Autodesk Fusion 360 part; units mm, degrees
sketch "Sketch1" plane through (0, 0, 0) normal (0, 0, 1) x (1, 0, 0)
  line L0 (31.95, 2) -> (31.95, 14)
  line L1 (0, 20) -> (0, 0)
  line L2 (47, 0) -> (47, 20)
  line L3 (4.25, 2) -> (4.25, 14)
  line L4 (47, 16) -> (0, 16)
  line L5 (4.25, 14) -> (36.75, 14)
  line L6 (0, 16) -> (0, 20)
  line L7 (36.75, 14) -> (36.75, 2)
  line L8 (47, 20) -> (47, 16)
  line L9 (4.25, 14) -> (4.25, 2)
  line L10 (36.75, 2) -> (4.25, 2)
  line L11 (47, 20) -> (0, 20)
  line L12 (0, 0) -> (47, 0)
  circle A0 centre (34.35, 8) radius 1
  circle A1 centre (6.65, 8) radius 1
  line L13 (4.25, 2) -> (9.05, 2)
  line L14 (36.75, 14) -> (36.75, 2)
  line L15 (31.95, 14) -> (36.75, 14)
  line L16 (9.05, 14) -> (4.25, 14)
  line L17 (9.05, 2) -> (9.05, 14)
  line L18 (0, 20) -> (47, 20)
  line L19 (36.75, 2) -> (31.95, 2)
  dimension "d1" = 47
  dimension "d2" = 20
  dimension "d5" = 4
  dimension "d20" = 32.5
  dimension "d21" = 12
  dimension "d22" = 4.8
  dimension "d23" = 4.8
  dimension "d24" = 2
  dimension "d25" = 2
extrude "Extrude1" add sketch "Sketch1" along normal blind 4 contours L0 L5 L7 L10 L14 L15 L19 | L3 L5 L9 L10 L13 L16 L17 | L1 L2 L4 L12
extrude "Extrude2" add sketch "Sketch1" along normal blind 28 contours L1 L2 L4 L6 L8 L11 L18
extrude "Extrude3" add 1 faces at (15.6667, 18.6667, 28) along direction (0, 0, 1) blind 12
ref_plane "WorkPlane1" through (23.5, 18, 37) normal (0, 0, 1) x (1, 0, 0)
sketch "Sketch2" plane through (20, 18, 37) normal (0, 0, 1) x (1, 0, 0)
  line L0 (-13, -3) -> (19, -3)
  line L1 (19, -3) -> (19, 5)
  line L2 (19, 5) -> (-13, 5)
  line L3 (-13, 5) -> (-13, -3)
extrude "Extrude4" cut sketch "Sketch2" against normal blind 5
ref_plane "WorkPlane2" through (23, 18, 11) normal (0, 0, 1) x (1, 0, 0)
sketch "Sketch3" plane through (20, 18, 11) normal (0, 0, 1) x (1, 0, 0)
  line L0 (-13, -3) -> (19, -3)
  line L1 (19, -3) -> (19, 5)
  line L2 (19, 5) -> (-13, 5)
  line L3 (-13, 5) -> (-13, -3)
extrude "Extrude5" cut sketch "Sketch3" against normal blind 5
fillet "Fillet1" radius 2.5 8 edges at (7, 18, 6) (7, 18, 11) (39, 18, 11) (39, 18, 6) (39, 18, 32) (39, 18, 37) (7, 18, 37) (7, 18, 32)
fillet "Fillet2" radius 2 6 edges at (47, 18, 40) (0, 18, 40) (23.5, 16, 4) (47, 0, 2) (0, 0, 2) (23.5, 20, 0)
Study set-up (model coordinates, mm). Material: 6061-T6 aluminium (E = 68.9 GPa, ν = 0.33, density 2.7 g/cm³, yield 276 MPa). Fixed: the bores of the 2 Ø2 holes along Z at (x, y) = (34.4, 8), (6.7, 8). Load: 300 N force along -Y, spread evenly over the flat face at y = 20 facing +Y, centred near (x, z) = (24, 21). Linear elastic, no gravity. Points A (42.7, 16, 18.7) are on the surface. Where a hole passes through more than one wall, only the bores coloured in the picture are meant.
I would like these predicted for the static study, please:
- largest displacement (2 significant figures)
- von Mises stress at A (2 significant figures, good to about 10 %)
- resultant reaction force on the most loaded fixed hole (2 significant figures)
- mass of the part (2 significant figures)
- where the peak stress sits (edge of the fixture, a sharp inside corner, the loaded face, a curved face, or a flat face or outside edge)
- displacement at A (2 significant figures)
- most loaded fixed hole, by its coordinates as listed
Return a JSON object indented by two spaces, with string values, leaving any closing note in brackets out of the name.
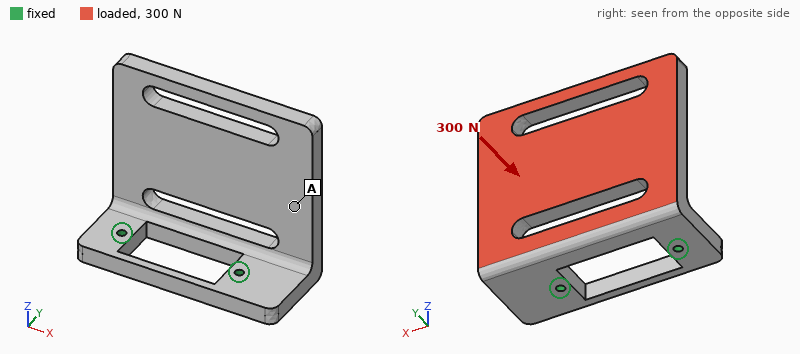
{
  "largest displacement": "0.52 mm",
  "von Mises stress at A": "25 MPa",
  "resultant reaction force on the most loaded fixed hole": "170 N",
  "mass of the part": "22 g",
  "where the peak stress sits": "a flat face or outside edge",
  "displacement at A": "0.18 mm",
  "most loaded fixed hole, by its coordinates as listed": "(34.4, 8)"
}
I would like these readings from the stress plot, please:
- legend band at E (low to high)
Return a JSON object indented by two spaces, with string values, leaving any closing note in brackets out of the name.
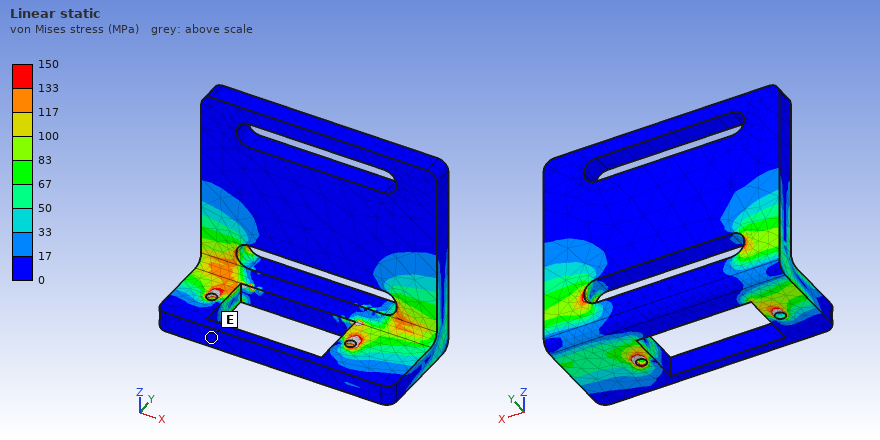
{
  "legend band at E": "0 to 17 MPa"
}
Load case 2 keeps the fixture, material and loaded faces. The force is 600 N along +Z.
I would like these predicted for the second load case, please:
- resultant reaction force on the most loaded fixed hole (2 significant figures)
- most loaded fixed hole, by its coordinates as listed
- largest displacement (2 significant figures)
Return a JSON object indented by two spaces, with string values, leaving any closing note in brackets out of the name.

{
  "resultant reaction force on the most loaded fixed hole": "350 N",
  "most loaded fixed hole, by its coordinates as listed": "(34.4, 8)",
  "largest displacement": "0.31 mm"
}
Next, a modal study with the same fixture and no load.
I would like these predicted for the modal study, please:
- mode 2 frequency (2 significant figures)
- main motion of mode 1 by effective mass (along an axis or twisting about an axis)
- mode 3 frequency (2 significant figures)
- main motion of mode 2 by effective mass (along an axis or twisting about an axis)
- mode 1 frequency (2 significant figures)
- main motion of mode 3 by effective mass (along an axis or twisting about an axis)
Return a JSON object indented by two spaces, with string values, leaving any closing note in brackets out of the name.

{
  "mode 2 frequency": "3200 Hz",
  "main motion of mode 1 by effective mass": "along Y",
  "mode 3 frequency": "4200 Hz",
  "main motion of mode 2 by effective mass": "along X",
  "mode 1 frequency": "1200 Hz",
  "main motion of mode 3 by effective mass": "along X"
}
